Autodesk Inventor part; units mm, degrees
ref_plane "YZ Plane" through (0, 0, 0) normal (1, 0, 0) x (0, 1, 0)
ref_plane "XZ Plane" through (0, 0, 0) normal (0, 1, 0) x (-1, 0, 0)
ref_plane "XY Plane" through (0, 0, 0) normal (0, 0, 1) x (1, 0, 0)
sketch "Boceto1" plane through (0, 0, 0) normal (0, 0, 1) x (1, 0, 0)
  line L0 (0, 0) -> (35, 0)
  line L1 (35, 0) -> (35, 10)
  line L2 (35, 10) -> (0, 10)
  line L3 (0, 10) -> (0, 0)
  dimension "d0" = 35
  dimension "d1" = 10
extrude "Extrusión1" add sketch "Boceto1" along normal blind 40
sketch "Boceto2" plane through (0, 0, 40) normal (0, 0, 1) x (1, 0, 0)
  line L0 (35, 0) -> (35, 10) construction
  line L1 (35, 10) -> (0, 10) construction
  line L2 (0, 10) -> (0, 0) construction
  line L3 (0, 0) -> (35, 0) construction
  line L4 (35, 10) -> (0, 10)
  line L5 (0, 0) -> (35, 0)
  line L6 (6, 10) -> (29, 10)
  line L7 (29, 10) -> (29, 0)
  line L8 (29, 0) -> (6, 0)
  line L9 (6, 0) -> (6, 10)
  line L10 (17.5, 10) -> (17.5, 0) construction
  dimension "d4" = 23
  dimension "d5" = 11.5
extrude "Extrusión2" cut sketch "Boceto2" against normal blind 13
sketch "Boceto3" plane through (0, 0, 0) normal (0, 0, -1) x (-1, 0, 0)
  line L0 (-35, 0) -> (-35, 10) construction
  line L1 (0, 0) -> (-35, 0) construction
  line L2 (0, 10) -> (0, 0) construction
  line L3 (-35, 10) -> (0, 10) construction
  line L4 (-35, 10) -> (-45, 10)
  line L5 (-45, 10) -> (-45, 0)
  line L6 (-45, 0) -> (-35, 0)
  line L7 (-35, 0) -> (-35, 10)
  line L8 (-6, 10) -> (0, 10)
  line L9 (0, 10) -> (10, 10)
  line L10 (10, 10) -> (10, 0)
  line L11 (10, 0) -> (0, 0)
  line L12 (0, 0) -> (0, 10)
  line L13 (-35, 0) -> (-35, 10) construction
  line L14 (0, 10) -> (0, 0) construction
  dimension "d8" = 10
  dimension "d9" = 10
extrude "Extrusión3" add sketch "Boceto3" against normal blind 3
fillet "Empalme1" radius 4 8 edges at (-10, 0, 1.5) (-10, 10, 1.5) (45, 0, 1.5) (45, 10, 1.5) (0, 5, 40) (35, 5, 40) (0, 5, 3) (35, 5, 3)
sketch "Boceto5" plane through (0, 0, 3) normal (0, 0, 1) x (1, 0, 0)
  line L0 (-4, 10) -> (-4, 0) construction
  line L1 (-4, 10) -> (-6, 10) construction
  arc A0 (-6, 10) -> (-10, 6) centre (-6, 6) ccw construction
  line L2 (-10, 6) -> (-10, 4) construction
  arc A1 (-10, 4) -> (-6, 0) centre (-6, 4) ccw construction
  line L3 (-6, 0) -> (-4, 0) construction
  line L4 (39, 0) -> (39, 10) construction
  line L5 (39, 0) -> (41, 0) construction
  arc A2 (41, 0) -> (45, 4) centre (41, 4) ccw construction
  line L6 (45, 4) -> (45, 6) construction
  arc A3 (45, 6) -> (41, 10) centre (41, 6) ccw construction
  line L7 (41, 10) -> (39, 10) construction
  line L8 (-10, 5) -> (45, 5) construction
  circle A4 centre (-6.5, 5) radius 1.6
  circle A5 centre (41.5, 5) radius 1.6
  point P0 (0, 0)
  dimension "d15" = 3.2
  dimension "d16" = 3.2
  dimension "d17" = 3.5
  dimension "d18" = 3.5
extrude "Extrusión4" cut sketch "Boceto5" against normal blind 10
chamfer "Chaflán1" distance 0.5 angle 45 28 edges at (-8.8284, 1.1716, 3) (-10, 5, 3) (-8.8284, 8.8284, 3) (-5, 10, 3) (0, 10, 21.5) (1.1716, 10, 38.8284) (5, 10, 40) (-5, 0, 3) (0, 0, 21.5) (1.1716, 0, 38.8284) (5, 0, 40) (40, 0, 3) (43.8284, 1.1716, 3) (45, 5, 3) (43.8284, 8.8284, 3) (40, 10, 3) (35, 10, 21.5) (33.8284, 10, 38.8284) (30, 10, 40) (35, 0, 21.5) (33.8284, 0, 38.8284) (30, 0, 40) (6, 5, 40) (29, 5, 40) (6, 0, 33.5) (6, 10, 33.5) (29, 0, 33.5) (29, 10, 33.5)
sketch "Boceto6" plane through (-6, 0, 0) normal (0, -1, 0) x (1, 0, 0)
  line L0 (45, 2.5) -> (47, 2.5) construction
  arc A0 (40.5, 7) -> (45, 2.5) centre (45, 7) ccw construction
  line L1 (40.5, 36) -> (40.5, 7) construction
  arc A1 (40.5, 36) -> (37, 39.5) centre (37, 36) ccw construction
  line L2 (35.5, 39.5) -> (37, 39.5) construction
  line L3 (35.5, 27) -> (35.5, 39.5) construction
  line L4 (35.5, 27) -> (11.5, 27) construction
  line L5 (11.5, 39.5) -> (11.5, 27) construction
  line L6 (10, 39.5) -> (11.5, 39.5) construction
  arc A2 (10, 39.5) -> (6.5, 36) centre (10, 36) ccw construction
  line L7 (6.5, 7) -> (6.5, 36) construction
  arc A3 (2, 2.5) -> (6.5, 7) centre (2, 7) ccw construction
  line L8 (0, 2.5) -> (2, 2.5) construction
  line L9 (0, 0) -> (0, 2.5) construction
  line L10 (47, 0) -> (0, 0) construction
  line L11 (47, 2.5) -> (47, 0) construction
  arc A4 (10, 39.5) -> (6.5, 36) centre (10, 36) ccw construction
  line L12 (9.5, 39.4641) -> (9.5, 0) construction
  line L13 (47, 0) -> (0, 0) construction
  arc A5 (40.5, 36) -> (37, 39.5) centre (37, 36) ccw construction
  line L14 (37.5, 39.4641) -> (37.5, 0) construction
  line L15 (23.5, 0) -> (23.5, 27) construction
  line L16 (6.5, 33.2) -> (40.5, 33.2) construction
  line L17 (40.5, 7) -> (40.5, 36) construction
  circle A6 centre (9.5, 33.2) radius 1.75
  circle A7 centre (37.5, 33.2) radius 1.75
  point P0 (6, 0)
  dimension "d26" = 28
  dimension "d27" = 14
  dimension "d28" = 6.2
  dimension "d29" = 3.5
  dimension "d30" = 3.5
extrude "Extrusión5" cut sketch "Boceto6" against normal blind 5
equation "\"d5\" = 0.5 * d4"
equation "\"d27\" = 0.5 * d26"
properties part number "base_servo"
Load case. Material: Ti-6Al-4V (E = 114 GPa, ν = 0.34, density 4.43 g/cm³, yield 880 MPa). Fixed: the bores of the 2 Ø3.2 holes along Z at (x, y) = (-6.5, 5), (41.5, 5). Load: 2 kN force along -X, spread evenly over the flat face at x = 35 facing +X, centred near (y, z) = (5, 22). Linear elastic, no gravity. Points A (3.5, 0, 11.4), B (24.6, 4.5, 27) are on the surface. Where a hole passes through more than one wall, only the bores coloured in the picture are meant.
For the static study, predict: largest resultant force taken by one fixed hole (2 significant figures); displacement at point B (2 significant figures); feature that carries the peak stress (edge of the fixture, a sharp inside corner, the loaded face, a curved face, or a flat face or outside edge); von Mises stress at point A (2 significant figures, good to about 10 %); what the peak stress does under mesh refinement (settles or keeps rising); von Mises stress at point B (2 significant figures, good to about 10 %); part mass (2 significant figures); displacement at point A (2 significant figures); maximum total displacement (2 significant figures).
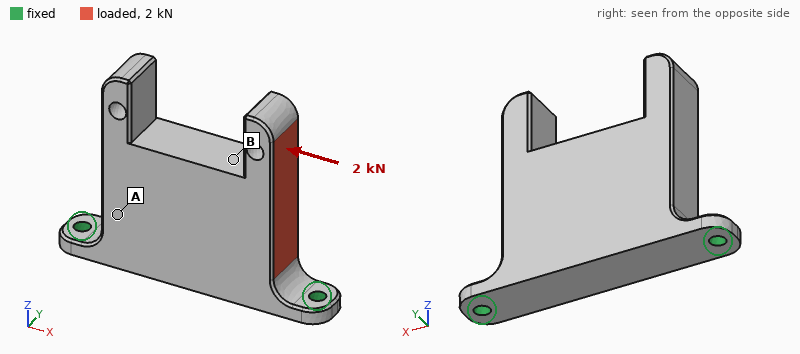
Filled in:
1.4 kN
19 µm
edge of the fixture
16 MPa
keeps rising
26 MPa
50 g
11 µm
46 µm
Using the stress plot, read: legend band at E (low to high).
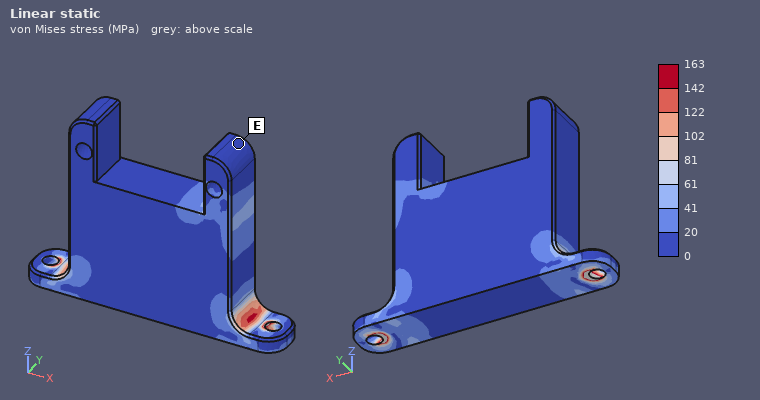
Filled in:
0 to 20 MPa
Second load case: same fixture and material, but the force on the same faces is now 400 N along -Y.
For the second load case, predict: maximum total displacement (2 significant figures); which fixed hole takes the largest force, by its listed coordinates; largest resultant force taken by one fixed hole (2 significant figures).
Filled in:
0.21 mm
(41.5, 5)
360 N
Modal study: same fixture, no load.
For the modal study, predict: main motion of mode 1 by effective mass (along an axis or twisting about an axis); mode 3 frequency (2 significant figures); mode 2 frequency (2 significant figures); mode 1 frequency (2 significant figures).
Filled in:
along Y
8600 Hz
8300 Hz
1600 Hz
